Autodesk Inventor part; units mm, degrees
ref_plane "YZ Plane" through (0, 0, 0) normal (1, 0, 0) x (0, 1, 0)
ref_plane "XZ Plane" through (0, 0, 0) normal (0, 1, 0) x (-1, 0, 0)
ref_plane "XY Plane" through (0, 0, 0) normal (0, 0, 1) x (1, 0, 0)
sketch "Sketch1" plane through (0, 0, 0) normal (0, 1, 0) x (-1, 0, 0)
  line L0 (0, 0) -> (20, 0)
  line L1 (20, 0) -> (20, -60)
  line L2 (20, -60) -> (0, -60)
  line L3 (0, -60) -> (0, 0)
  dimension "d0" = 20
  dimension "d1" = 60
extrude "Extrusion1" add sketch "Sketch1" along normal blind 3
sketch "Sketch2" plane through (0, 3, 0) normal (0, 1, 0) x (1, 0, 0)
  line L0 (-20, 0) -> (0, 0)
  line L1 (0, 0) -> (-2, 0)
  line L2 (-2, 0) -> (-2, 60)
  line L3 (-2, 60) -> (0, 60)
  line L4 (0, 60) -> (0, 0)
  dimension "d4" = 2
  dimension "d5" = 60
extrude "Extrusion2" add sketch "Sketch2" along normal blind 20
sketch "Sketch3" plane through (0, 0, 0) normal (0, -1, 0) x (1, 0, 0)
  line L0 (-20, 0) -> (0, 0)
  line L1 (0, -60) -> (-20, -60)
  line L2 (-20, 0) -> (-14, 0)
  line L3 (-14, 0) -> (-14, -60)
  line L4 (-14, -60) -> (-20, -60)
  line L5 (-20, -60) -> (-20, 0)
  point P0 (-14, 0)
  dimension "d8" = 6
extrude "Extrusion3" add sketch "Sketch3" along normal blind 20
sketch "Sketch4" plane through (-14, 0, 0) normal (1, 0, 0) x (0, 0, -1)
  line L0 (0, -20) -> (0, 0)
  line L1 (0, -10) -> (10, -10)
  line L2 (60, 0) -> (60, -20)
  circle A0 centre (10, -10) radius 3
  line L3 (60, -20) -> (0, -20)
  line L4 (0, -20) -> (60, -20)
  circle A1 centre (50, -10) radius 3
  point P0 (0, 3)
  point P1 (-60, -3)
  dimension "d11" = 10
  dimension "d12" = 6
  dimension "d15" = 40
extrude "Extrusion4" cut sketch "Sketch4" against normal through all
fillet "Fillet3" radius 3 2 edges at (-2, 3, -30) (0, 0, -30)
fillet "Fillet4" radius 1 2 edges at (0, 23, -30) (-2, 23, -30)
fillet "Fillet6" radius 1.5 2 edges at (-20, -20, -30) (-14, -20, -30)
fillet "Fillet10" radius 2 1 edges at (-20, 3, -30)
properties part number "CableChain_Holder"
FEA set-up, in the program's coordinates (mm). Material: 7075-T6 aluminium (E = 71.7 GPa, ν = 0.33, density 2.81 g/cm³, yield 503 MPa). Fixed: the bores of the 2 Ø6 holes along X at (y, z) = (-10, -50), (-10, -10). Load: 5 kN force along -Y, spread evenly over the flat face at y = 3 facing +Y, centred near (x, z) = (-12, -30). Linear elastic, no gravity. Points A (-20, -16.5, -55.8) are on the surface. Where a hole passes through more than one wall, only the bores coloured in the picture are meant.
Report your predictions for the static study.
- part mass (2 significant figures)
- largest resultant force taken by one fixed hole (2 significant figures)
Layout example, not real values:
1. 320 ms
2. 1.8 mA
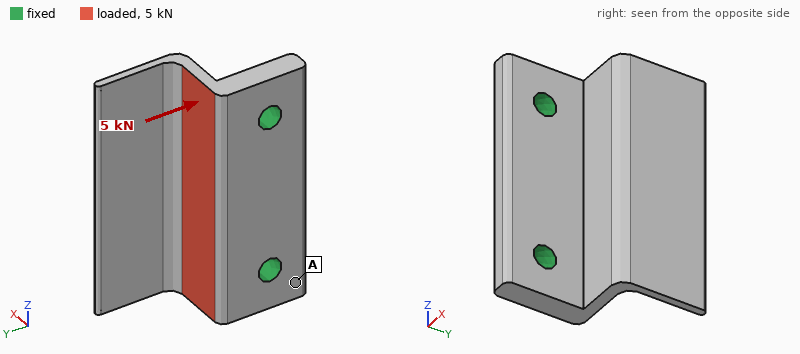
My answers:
1. 36 g
2. 2.5 kN
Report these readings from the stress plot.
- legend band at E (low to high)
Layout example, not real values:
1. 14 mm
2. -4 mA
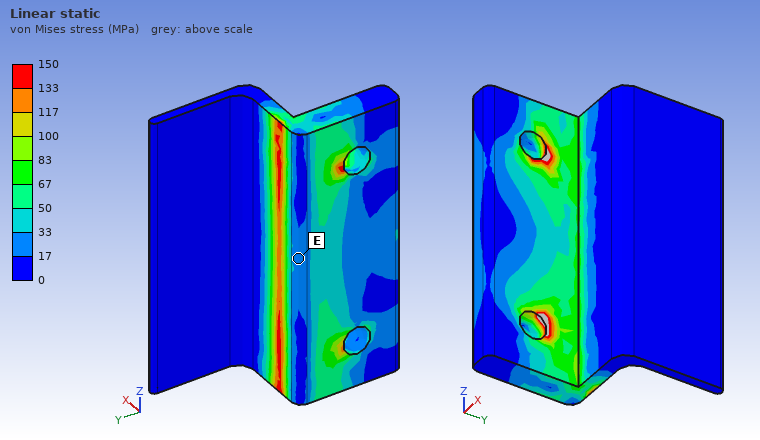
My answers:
1. 17 to 33 MPa
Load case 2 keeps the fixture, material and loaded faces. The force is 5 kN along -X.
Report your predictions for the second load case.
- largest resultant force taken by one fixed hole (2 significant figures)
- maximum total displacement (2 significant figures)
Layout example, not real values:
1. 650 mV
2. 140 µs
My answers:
1. 2.5 kN
2. 0.29 mm
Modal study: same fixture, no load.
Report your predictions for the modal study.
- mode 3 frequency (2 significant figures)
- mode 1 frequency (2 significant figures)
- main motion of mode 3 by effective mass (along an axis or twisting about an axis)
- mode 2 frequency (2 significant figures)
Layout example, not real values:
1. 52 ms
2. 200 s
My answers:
1. 6900 Hz
2. 2700 Hz
3. along Y
4. 3800 Hz
